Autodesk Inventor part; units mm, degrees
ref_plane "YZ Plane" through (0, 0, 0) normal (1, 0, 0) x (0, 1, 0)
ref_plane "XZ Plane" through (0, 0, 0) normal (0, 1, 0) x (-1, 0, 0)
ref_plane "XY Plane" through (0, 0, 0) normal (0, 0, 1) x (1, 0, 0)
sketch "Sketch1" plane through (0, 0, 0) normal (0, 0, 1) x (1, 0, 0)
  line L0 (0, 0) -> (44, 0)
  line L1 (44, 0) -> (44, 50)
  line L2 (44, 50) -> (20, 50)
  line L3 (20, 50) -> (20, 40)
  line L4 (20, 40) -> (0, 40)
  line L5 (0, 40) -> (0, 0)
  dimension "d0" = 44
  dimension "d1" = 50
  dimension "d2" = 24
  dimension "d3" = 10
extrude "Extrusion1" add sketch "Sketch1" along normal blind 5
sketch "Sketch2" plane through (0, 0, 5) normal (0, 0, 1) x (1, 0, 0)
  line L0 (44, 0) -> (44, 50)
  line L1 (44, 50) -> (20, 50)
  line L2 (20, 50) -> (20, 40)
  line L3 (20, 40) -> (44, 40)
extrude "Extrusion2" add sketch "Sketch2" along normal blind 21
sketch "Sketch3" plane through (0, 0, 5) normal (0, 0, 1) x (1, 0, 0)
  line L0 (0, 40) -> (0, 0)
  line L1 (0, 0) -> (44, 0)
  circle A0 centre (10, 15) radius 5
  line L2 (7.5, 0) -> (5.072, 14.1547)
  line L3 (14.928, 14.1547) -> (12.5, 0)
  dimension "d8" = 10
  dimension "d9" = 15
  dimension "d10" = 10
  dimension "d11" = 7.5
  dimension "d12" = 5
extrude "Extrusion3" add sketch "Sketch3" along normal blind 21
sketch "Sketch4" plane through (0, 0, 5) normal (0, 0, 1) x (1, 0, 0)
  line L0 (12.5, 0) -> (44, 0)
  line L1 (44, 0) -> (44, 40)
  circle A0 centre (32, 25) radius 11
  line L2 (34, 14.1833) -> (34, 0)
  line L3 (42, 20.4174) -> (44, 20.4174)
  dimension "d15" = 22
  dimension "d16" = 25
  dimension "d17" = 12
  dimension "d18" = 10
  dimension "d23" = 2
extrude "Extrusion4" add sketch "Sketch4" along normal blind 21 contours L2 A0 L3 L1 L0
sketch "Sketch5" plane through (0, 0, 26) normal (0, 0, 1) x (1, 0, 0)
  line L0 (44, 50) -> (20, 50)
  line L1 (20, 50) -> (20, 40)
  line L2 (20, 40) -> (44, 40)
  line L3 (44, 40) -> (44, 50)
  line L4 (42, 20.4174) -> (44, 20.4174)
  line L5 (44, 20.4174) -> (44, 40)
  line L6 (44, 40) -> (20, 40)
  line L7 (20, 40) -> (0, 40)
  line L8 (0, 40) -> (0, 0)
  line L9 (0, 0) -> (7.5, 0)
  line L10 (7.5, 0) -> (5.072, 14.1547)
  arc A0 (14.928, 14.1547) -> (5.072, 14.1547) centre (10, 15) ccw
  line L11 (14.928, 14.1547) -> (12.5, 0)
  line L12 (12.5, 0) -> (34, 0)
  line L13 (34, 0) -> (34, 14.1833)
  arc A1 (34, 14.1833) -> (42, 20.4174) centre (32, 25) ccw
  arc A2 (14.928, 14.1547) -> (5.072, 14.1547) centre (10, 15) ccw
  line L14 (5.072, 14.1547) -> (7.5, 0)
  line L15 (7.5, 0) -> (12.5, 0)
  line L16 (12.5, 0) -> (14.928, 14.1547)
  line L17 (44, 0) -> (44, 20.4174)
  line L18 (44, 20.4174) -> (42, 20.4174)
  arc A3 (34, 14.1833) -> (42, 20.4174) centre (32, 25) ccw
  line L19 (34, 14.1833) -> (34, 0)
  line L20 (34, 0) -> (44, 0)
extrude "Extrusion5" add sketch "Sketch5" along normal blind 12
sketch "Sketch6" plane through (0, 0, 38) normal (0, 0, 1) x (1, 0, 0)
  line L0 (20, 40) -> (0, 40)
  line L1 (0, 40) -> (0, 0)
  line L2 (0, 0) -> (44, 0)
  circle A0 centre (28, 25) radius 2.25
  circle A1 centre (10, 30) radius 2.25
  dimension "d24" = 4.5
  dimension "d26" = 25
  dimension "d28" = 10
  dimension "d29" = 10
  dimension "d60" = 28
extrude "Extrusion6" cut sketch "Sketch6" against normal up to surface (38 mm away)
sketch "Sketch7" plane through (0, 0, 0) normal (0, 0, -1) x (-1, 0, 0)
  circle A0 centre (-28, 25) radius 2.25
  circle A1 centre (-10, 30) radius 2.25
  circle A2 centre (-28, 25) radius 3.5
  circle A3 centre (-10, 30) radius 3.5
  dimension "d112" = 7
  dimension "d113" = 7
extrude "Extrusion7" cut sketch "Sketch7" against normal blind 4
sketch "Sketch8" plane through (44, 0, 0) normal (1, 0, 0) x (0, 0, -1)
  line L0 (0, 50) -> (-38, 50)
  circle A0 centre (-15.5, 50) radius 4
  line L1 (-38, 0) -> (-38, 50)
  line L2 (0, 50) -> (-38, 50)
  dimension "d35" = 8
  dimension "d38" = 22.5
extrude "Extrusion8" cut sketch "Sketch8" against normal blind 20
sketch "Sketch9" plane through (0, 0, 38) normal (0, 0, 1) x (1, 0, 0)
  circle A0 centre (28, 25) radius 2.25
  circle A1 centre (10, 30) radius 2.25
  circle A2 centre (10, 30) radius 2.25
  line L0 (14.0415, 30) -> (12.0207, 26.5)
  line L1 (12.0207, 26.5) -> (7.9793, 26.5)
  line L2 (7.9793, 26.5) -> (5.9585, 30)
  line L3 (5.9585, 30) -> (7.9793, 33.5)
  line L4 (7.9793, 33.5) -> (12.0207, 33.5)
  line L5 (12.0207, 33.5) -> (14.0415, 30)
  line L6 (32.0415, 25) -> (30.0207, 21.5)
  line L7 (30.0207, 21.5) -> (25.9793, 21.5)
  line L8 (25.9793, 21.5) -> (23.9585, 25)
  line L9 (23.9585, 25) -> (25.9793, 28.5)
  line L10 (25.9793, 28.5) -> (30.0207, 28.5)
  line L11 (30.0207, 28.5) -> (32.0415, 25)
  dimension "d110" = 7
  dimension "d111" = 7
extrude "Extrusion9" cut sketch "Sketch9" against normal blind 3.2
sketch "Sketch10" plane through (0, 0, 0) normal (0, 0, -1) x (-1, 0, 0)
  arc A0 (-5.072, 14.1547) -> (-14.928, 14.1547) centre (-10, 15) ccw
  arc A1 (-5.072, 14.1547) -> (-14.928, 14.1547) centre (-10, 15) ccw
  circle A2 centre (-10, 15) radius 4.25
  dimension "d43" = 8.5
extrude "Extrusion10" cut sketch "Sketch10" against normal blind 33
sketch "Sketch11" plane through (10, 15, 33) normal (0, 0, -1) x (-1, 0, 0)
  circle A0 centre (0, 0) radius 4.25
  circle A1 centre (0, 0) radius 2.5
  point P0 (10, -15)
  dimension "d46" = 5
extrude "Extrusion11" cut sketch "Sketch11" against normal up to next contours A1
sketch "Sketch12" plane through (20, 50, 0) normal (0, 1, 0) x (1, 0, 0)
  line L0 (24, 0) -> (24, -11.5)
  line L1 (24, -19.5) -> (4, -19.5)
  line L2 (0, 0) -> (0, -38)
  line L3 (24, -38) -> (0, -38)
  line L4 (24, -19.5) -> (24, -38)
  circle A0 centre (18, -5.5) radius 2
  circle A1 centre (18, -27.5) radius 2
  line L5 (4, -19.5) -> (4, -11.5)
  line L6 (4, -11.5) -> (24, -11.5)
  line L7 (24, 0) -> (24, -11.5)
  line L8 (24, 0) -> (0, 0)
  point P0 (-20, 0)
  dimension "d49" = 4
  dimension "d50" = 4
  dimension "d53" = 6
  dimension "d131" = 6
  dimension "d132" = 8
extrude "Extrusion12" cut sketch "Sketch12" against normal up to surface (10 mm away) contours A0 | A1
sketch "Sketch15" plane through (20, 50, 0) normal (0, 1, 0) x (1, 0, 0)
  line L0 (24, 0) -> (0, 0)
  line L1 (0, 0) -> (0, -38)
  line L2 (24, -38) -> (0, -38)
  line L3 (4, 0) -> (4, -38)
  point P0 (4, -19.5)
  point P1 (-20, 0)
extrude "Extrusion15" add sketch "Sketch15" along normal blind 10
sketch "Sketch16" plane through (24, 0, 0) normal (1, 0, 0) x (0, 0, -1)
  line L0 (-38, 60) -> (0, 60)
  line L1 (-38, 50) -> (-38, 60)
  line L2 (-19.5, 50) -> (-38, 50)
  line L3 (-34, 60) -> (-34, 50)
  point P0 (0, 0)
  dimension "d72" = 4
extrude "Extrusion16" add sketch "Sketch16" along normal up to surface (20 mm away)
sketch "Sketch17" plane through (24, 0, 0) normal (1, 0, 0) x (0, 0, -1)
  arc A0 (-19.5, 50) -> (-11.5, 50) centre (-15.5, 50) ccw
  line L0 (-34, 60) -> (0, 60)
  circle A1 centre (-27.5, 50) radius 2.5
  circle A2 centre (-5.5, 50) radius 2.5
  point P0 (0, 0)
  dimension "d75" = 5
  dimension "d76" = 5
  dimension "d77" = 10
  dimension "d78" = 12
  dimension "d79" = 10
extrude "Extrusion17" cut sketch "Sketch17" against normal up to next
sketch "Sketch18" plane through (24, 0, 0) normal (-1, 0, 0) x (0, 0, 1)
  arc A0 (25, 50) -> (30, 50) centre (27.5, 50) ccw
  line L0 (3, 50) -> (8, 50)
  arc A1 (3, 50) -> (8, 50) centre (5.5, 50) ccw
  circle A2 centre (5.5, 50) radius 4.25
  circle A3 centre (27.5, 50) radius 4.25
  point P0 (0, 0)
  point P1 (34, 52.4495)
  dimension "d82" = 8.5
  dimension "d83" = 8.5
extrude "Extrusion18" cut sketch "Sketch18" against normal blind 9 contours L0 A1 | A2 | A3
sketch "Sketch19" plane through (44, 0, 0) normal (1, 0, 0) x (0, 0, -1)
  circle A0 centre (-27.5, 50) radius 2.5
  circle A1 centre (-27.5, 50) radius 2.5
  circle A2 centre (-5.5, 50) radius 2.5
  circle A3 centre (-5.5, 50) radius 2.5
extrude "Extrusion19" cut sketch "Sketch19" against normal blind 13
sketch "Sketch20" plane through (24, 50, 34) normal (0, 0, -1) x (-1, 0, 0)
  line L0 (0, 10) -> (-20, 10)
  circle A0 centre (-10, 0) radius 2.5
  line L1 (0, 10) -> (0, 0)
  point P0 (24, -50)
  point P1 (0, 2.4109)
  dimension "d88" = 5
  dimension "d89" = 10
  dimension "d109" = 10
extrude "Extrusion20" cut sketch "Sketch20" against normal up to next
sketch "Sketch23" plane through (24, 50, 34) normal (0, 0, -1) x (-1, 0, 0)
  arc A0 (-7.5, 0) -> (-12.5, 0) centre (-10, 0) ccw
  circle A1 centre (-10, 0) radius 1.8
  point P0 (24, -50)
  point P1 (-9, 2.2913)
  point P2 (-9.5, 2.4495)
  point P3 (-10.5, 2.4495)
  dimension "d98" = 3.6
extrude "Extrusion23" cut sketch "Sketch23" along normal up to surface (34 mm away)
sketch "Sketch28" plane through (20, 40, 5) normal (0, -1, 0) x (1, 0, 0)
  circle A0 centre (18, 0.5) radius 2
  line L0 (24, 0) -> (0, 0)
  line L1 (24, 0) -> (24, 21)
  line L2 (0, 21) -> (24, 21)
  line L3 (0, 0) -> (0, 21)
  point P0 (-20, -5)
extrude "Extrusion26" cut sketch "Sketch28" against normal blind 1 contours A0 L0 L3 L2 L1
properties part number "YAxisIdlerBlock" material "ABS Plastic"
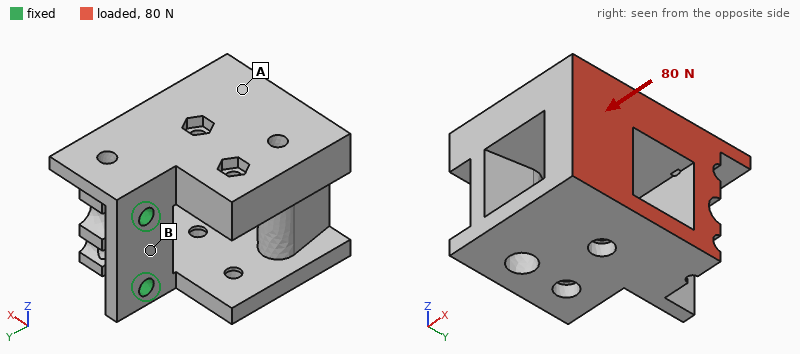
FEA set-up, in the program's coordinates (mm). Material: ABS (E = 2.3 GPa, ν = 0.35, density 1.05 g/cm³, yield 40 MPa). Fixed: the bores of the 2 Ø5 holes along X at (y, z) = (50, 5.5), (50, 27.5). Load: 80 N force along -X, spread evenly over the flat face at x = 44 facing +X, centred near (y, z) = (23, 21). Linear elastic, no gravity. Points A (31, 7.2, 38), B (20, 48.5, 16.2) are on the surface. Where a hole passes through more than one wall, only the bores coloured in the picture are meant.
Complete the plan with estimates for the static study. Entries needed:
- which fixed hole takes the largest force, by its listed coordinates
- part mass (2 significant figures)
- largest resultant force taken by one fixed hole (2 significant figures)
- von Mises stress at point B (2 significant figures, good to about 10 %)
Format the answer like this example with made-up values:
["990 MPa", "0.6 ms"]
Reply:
["(50, 27.5)", "45 g", "56 N", "4.3 MPa"]
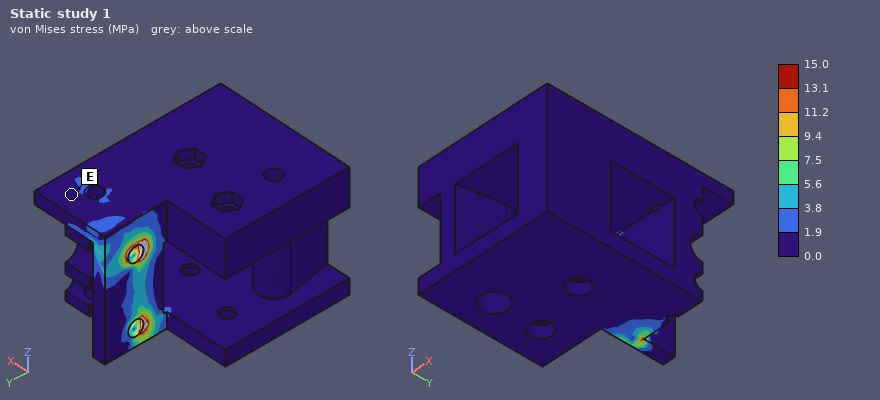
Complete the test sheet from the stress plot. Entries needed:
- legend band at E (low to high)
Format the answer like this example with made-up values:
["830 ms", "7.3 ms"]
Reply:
["0.0 to 1.9 MPa"]
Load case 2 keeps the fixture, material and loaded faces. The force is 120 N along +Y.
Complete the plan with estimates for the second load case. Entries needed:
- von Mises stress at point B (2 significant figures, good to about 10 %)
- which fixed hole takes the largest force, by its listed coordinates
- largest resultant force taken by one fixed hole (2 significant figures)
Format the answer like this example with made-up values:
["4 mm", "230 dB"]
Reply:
["5.9 MPa", "(50, 27.5)", "77 N"]
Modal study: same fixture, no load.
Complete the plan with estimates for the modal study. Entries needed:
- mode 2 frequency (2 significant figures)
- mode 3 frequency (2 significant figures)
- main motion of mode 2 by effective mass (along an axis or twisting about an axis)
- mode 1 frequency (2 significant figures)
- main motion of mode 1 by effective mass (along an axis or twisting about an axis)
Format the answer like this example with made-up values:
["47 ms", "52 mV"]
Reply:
["750 Hz", "1200 Hz", "along Z", "300 Hz", "along X"]
